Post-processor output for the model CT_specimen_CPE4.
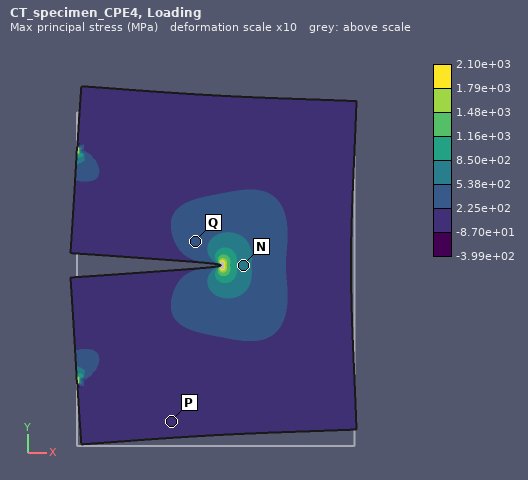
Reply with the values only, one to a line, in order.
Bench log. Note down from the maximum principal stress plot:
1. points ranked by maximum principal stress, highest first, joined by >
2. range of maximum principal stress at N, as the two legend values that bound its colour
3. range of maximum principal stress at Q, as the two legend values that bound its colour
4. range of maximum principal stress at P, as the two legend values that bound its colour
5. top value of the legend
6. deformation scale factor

N > Q > P
5.38e+02 to 8.50e+02 MPa
2.25e+02 to 5.38e+02 MPa
-8.70e+01 to 2.25e+02 MPa
2.10e+03 MPa
10
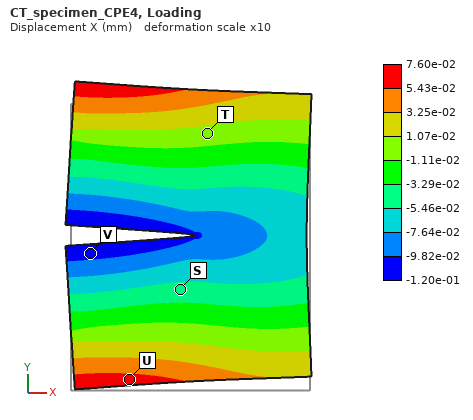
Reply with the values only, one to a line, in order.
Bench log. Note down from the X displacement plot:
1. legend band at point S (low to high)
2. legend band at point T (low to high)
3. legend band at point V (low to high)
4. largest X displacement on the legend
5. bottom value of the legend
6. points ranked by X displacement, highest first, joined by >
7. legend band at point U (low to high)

-5.46e-02 to -3.29e-02 mm
-1.11e-02 to 1.07e-02 mm
-1.20e-01 to -9.82e-02 mm
7.60e-02 mm
-1.20e-01 mm
U > T > S > V
5.43e-02 to 7.60e-02 mm
